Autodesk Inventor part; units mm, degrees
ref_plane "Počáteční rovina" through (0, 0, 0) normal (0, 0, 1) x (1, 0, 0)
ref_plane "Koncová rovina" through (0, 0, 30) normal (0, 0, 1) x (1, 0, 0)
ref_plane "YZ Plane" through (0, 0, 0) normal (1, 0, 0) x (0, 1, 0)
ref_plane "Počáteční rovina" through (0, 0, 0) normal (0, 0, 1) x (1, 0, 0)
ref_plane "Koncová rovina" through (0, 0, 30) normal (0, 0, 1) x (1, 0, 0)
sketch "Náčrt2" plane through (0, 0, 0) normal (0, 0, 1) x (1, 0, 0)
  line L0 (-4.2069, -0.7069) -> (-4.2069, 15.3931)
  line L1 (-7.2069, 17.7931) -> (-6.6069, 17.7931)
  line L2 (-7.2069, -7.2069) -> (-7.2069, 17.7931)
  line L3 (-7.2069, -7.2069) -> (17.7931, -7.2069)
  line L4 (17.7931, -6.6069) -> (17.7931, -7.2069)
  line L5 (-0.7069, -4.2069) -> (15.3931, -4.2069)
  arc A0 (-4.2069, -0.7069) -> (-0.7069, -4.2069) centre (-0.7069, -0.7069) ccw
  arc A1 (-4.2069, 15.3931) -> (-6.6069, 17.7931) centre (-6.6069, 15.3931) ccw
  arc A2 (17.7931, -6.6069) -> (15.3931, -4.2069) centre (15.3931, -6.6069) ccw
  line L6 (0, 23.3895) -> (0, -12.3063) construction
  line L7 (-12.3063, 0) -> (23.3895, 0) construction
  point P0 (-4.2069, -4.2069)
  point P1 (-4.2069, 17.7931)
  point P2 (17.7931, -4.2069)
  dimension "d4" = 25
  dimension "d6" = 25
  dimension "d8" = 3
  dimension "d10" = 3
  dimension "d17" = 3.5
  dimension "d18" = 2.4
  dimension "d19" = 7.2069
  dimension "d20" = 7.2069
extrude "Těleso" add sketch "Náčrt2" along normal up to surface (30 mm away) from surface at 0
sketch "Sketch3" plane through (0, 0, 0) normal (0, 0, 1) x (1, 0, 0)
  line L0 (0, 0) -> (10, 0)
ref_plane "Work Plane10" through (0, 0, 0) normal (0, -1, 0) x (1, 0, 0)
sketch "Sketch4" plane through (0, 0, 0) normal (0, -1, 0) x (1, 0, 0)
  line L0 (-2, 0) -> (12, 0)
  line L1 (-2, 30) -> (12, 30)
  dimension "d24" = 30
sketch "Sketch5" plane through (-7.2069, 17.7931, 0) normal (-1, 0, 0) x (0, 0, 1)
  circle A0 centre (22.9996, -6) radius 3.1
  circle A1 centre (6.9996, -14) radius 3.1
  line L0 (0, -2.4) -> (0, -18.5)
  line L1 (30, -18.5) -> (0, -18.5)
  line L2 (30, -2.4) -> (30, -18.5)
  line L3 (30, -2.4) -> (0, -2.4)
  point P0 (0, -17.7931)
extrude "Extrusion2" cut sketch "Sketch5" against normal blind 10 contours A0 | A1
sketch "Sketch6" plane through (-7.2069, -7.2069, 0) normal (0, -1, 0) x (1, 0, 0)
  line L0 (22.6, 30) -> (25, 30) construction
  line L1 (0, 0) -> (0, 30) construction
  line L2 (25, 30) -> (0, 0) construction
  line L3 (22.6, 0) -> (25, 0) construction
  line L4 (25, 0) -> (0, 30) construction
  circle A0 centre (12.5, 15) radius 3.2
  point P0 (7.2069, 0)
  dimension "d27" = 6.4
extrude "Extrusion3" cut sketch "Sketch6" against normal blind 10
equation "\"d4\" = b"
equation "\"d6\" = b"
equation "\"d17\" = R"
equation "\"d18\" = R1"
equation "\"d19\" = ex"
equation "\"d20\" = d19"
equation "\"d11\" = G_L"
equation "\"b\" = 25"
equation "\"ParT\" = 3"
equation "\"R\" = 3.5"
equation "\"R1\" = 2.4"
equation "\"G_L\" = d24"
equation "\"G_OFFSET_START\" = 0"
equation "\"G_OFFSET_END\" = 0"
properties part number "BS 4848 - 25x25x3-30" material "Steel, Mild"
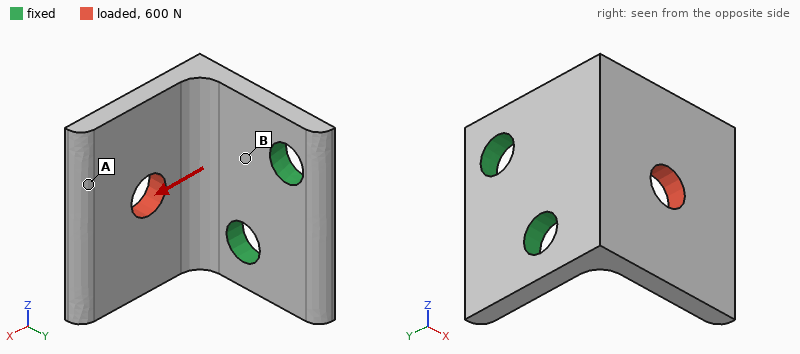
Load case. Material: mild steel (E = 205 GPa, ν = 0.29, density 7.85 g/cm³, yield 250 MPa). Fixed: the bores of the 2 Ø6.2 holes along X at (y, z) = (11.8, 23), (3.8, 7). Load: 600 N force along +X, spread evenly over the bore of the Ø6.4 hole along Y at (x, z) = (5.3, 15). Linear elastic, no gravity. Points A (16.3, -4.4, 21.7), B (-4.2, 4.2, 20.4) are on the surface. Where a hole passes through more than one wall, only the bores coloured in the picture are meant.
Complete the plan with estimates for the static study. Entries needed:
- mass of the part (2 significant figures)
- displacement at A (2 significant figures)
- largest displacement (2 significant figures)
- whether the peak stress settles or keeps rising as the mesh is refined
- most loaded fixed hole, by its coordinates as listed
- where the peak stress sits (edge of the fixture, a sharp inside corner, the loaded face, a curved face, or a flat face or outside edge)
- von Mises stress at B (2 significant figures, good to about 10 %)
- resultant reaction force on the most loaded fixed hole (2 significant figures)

31 g
50 µm
59 µm
keeps rising
(3.8, 7)
edge of the fixture
59 MPa
480 N
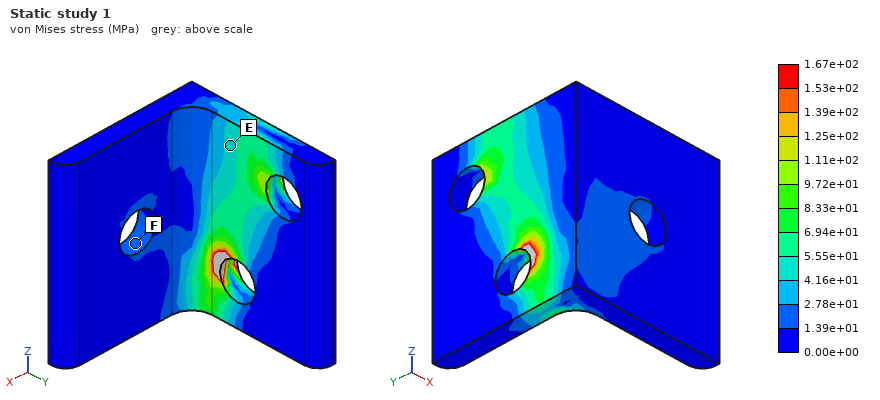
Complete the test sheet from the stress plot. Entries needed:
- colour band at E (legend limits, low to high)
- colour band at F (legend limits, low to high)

4.16e+01 to 5.55e+01 MPa
1.39e+01 to 2.78e+01 MPa
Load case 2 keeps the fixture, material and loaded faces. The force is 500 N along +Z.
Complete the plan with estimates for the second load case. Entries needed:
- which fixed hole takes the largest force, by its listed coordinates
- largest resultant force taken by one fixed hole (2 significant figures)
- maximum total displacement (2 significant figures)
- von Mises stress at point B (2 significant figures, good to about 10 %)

(3.8, 7)
510 N
36 µm
41 MPa
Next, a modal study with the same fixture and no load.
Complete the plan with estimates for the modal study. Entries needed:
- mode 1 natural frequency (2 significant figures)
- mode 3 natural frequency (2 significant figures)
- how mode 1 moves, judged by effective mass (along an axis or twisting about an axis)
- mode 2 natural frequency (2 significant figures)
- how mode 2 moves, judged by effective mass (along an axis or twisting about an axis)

3200 Hz
8900 Hz
along Y
5700 Hz
along Z
